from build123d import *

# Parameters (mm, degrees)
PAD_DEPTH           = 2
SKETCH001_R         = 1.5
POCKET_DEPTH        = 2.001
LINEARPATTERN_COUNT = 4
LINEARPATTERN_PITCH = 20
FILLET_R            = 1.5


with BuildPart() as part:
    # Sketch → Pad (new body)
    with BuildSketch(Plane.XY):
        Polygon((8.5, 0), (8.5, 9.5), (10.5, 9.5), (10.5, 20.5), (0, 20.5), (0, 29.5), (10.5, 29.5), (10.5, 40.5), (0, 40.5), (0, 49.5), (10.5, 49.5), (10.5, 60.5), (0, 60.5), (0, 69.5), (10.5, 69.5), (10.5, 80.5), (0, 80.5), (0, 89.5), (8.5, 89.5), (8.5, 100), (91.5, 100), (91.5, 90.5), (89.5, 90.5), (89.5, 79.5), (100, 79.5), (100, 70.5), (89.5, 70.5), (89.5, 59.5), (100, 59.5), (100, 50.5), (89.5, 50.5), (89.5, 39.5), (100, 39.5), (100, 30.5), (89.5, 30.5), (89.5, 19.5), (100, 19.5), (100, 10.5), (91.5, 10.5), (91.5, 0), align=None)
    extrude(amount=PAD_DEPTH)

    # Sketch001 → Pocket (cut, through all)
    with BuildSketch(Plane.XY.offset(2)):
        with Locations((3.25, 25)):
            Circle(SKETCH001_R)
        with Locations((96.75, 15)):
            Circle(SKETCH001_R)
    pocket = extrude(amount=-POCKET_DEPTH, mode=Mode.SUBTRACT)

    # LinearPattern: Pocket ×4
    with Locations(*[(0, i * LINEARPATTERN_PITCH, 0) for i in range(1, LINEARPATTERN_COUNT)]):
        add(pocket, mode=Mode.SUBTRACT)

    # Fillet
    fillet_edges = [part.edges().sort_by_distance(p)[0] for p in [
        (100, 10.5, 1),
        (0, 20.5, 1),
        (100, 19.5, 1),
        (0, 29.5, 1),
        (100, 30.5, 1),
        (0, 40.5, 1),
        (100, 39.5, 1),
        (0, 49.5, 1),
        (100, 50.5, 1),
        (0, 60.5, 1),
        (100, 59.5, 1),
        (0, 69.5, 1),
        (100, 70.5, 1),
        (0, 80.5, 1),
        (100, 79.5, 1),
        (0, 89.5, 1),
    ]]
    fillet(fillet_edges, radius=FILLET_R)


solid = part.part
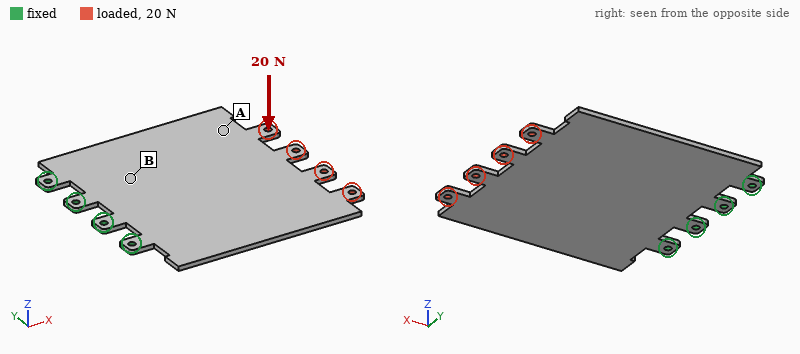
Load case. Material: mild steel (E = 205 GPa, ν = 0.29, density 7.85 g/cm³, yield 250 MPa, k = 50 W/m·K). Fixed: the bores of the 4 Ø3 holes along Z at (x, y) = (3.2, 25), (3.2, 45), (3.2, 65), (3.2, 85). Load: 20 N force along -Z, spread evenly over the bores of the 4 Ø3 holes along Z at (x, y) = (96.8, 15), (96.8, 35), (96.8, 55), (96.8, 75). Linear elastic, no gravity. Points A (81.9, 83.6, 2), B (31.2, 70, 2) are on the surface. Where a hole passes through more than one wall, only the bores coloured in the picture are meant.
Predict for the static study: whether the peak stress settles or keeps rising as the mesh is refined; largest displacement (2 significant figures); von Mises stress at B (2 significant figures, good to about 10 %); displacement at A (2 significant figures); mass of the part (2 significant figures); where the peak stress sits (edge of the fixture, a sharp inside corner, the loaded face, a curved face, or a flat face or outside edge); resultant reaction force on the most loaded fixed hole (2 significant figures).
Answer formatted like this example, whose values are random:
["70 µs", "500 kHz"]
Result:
["keeps rising", "0.61 mm", "20 MPa", "0.41 mm", "140 g", "edge of the fixture", "9.6 N"]
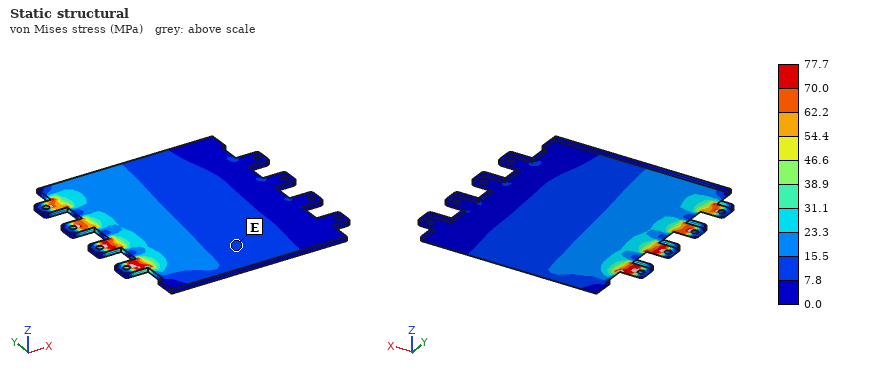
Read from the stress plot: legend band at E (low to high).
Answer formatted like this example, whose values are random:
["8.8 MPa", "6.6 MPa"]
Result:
["7.8 to 15.5 MPa"]
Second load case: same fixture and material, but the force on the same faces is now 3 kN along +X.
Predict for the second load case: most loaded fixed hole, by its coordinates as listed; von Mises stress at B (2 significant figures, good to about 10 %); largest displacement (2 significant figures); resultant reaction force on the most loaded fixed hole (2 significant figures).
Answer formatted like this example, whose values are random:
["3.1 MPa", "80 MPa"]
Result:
["(3.2, 25)", "14 MPa", "18 µm", "1.3 kN"]
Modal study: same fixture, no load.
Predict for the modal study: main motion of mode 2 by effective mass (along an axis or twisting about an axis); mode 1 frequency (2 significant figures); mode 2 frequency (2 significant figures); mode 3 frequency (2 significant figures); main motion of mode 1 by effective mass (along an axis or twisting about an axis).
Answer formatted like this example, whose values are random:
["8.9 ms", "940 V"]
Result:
["twisting about X", "160 Hz", "400 Hz", "1000 Hz", "along Z"]
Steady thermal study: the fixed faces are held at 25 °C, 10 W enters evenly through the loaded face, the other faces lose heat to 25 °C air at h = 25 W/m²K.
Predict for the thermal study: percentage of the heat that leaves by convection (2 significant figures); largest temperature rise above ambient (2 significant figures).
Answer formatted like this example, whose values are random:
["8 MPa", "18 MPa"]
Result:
["82 %", "69 K"]
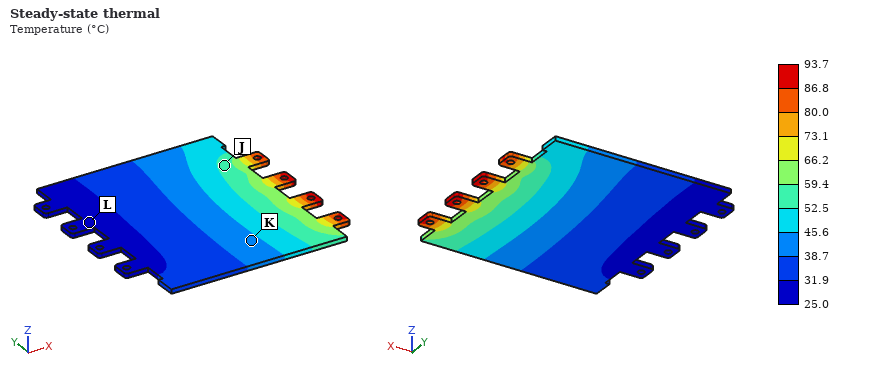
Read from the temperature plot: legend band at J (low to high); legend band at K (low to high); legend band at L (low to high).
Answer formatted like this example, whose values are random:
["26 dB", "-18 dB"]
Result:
["52.5 to 59.4 °C", "38.7 to 45.6 °C", "25.0 to 31.9 °C"]
